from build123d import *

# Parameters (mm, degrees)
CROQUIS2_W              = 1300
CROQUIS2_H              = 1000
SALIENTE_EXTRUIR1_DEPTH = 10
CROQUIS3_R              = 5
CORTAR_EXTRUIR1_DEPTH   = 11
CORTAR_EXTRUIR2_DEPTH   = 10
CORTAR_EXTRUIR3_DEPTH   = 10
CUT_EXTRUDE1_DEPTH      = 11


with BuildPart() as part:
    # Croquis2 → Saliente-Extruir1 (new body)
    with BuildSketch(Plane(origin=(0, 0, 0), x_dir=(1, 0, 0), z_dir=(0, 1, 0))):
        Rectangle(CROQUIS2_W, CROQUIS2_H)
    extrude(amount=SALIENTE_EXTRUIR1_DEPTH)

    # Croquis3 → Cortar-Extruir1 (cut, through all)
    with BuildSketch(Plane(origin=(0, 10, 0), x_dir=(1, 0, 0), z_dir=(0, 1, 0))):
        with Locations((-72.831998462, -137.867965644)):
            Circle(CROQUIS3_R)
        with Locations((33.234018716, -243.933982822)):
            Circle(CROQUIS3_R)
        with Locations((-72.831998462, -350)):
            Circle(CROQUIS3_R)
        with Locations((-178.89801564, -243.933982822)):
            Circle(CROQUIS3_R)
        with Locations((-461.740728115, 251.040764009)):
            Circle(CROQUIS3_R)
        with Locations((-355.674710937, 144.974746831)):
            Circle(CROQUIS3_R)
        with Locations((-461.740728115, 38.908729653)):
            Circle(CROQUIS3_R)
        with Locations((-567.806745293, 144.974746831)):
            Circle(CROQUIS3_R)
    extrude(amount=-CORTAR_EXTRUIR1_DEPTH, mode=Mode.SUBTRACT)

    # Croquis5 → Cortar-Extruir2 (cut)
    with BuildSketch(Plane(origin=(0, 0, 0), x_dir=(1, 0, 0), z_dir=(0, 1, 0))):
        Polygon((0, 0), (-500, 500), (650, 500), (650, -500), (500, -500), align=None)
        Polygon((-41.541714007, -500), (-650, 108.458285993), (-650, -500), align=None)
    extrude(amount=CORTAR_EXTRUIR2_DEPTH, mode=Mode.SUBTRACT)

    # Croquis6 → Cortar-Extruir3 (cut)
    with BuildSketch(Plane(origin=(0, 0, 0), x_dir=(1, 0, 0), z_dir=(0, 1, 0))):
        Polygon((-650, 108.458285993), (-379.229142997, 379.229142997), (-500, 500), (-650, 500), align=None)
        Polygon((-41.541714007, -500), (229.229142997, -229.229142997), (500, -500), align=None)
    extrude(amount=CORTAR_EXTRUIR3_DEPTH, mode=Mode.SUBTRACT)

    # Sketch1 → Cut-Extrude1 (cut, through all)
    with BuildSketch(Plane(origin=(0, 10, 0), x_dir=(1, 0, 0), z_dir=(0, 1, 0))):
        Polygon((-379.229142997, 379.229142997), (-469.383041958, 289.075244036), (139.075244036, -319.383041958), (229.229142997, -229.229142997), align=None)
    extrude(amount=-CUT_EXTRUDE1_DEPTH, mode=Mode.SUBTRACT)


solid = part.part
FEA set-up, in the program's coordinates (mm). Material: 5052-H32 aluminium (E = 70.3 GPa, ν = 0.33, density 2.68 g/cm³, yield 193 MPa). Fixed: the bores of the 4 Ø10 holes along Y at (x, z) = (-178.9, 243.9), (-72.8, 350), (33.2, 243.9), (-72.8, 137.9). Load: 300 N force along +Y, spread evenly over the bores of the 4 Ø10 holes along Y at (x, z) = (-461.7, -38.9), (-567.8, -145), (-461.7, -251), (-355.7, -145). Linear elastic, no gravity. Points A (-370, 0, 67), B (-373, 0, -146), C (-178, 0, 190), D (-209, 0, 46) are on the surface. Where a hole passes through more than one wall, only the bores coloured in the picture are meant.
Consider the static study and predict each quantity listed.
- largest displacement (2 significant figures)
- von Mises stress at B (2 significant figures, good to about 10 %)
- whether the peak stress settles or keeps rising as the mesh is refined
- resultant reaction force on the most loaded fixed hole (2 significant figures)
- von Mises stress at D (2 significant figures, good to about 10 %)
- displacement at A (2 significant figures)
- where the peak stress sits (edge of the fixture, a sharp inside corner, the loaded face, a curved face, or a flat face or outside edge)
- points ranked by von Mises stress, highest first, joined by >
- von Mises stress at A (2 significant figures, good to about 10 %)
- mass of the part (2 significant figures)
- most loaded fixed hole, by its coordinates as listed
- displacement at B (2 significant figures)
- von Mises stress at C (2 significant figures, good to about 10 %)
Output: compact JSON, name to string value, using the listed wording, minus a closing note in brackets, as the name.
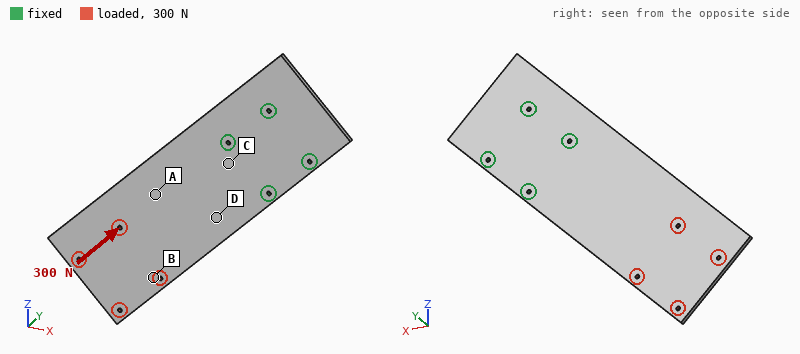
{"largest displacement": "10 mm", "von Mises stress at B": "5.5 MPa", "whether the peak stress settles or keeps rising as the mesh is refined": "keeps rising", "resultant reaction force on the most loaded fixed hole": "450 N", "von Mises stress at D": "22 MPa", "displacement at A": "2.7 mm", "where the peak stress sits": "edge of the fixture", "points ranked by von Mises stress, highest first, joined by >": "C > D > A > B", "von Mises stress at A": "15 MPa", "mass of the part": "5.9 kg", "most loaded fixed hole, by its coordinates as listed": "(-178.9, 243.9)", "displacement at B": "6.1 mm", "von Mises stress at C": "29 MPa"}
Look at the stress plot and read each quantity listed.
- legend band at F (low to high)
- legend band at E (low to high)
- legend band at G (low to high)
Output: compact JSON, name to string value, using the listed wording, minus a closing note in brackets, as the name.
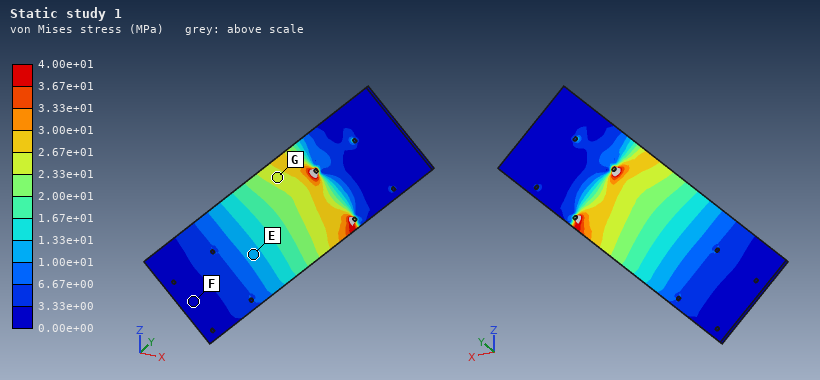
{"legend band at F": "0.00e+00 to 3.33e+00 MPa", "legend band at E": "1.00e+01 to 1.33e+01 MPa", "legend band at G": "2.33e+01 to 2.67e+01 MPa"}
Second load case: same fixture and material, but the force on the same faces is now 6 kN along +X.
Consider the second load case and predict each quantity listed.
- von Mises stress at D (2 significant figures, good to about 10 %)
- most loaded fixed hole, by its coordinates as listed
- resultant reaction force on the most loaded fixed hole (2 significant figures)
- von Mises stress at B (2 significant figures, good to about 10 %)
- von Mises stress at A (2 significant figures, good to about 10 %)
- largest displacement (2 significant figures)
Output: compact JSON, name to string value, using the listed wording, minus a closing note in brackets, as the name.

{"von Mises stress at D": "10 MPa", "most loaded fixed hole, by its coordinates as listed": "(-72.8, 137.9)", "resultant reaction force on the most loaded fixed hole": "12 kN", "von Mises stress at B": "5.0 MPa", "von Mises stress at A": "4.2 MPa", "largest displacement": "0.34 mm"}
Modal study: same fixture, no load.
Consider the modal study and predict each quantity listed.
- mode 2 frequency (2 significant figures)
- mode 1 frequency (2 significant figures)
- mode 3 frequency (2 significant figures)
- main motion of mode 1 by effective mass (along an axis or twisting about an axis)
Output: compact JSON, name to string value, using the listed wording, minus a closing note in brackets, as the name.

{"mode 2 frequency": "120 Hz", "mode 1 frequency": "24 Hz", "mode 3 frequency": "150 Hz", "main motion of mode 1 by effective mass": "along Y"}
